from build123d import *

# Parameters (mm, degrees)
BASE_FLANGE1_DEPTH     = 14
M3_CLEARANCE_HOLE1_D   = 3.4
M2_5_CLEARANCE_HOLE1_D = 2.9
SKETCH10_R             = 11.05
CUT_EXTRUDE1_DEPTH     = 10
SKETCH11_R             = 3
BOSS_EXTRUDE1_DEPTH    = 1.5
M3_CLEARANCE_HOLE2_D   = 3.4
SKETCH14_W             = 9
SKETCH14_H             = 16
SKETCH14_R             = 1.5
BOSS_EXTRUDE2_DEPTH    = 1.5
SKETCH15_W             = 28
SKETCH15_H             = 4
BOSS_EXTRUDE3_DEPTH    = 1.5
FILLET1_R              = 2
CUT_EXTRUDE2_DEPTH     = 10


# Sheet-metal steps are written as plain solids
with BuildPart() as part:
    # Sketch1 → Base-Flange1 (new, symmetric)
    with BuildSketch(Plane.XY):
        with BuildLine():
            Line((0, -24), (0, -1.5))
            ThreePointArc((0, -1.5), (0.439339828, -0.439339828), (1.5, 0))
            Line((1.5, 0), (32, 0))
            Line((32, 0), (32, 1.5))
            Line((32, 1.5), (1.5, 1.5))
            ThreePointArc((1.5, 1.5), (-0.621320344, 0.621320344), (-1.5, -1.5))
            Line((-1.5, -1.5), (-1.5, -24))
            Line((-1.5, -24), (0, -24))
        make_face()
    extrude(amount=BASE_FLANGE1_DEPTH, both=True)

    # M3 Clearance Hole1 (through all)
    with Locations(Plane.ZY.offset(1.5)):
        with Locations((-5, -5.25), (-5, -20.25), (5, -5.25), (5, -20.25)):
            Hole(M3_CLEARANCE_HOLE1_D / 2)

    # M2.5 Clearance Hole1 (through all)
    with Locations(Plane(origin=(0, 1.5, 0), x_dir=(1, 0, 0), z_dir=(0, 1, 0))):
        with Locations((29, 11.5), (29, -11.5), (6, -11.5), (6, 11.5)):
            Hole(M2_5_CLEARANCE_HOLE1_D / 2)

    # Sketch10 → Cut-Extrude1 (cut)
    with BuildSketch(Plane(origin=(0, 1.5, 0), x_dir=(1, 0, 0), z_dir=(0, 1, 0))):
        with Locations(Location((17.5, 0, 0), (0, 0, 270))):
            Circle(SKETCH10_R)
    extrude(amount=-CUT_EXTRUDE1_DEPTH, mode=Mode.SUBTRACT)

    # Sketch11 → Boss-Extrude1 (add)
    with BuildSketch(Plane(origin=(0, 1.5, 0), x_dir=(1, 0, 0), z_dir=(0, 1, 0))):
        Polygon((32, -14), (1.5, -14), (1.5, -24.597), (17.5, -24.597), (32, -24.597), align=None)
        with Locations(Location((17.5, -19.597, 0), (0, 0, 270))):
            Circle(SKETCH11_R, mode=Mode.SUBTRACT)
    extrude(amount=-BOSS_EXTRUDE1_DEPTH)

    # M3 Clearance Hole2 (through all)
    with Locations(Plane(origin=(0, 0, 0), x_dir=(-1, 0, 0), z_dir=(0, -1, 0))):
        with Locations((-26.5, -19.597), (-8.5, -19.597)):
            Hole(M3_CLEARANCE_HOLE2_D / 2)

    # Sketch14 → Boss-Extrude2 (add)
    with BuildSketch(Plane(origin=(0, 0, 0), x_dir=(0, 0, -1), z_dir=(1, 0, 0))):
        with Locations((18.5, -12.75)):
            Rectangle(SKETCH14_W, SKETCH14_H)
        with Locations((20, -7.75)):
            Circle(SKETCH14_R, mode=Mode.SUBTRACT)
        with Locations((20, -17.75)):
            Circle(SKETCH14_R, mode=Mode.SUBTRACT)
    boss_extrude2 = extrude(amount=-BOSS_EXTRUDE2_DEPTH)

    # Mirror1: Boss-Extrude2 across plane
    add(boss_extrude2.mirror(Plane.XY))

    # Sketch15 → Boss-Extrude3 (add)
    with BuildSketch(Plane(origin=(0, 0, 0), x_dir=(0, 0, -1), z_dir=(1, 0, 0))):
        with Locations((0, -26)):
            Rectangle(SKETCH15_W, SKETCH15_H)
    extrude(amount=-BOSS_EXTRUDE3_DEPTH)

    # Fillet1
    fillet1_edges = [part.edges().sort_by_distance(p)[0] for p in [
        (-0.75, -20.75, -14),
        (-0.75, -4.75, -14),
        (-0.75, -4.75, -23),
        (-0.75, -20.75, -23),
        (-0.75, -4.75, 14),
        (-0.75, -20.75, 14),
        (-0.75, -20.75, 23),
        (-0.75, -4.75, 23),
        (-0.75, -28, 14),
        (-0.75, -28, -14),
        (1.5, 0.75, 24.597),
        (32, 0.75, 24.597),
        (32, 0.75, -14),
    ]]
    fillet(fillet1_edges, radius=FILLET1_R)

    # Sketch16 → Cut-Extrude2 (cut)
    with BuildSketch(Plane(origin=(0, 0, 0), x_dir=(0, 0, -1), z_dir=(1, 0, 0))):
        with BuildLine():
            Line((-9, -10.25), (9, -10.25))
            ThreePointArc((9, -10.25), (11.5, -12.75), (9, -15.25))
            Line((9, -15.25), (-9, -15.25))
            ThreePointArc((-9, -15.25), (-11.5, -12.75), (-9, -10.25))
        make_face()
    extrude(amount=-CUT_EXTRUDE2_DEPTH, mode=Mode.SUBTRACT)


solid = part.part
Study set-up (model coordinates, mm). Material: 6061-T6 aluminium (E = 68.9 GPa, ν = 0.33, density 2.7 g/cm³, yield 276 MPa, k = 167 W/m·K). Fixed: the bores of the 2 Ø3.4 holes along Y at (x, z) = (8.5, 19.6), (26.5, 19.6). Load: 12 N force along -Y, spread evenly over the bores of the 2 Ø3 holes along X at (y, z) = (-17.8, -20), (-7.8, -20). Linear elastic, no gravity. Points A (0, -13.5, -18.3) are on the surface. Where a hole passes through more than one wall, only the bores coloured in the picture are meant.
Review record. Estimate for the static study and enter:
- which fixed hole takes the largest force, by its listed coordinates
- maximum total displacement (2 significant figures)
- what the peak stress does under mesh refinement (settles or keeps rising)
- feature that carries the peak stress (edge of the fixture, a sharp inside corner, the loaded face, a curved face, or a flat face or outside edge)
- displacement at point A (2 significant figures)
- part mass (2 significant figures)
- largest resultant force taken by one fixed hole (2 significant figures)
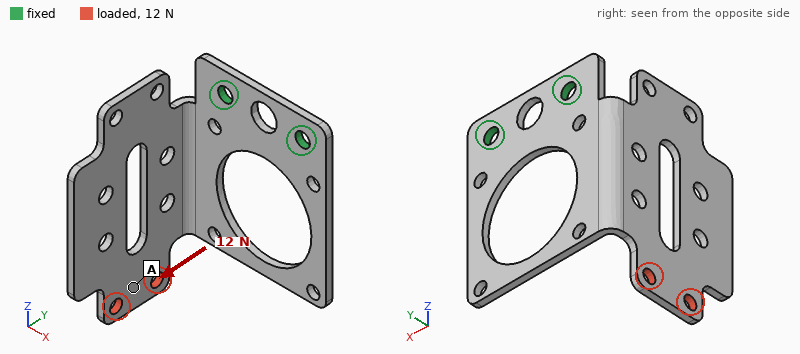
(8.5, 19.6)
0.78 mm
keeps rising
a sharp inside corner
0.65 mm
6.8 g
16 N
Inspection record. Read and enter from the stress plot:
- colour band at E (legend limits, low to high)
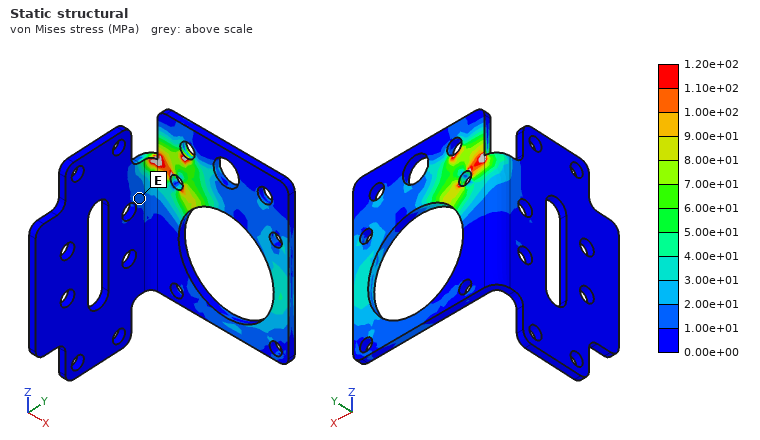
1.00e+01 to 2.00e+01 MPa
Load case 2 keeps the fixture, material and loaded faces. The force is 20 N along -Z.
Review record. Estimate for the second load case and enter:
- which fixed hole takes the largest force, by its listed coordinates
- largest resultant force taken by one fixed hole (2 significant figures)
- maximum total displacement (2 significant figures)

(8.5, 19.6)
27 N
0.48 mm
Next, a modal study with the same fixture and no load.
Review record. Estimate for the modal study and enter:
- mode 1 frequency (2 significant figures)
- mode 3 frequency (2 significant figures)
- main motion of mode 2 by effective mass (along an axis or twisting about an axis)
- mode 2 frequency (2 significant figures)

450 Hz
1800 Hz
along X
720 Hz
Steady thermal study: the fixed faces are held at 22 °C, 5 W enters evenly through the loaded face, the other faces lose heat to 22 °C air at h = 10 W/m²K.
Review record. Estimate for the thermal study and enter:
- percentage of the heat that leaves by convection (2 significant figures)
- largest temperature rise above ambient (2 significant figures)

18 %
53 K
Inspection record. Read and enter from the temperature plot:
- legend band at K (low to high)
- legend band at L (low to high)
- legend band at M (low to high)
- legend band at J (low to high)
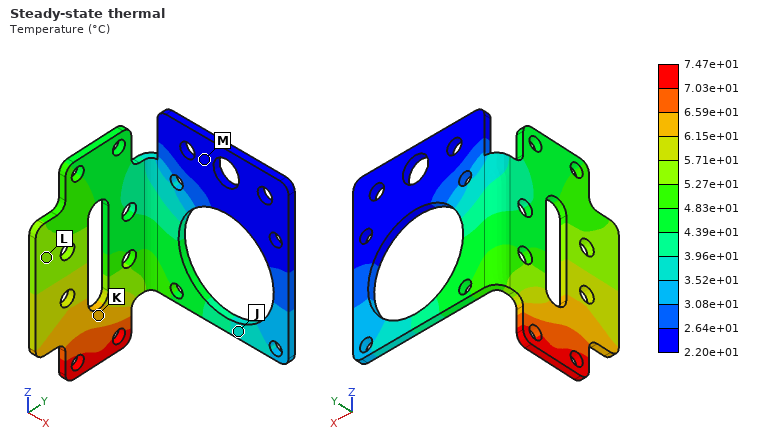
6.15e+01 to 6.59e+01 °C
5.27e+01 to 5.71e+01 °C
2.20e+01 to 2.64e+01 °C
3.52e+01 to 3.96e+01 °C
